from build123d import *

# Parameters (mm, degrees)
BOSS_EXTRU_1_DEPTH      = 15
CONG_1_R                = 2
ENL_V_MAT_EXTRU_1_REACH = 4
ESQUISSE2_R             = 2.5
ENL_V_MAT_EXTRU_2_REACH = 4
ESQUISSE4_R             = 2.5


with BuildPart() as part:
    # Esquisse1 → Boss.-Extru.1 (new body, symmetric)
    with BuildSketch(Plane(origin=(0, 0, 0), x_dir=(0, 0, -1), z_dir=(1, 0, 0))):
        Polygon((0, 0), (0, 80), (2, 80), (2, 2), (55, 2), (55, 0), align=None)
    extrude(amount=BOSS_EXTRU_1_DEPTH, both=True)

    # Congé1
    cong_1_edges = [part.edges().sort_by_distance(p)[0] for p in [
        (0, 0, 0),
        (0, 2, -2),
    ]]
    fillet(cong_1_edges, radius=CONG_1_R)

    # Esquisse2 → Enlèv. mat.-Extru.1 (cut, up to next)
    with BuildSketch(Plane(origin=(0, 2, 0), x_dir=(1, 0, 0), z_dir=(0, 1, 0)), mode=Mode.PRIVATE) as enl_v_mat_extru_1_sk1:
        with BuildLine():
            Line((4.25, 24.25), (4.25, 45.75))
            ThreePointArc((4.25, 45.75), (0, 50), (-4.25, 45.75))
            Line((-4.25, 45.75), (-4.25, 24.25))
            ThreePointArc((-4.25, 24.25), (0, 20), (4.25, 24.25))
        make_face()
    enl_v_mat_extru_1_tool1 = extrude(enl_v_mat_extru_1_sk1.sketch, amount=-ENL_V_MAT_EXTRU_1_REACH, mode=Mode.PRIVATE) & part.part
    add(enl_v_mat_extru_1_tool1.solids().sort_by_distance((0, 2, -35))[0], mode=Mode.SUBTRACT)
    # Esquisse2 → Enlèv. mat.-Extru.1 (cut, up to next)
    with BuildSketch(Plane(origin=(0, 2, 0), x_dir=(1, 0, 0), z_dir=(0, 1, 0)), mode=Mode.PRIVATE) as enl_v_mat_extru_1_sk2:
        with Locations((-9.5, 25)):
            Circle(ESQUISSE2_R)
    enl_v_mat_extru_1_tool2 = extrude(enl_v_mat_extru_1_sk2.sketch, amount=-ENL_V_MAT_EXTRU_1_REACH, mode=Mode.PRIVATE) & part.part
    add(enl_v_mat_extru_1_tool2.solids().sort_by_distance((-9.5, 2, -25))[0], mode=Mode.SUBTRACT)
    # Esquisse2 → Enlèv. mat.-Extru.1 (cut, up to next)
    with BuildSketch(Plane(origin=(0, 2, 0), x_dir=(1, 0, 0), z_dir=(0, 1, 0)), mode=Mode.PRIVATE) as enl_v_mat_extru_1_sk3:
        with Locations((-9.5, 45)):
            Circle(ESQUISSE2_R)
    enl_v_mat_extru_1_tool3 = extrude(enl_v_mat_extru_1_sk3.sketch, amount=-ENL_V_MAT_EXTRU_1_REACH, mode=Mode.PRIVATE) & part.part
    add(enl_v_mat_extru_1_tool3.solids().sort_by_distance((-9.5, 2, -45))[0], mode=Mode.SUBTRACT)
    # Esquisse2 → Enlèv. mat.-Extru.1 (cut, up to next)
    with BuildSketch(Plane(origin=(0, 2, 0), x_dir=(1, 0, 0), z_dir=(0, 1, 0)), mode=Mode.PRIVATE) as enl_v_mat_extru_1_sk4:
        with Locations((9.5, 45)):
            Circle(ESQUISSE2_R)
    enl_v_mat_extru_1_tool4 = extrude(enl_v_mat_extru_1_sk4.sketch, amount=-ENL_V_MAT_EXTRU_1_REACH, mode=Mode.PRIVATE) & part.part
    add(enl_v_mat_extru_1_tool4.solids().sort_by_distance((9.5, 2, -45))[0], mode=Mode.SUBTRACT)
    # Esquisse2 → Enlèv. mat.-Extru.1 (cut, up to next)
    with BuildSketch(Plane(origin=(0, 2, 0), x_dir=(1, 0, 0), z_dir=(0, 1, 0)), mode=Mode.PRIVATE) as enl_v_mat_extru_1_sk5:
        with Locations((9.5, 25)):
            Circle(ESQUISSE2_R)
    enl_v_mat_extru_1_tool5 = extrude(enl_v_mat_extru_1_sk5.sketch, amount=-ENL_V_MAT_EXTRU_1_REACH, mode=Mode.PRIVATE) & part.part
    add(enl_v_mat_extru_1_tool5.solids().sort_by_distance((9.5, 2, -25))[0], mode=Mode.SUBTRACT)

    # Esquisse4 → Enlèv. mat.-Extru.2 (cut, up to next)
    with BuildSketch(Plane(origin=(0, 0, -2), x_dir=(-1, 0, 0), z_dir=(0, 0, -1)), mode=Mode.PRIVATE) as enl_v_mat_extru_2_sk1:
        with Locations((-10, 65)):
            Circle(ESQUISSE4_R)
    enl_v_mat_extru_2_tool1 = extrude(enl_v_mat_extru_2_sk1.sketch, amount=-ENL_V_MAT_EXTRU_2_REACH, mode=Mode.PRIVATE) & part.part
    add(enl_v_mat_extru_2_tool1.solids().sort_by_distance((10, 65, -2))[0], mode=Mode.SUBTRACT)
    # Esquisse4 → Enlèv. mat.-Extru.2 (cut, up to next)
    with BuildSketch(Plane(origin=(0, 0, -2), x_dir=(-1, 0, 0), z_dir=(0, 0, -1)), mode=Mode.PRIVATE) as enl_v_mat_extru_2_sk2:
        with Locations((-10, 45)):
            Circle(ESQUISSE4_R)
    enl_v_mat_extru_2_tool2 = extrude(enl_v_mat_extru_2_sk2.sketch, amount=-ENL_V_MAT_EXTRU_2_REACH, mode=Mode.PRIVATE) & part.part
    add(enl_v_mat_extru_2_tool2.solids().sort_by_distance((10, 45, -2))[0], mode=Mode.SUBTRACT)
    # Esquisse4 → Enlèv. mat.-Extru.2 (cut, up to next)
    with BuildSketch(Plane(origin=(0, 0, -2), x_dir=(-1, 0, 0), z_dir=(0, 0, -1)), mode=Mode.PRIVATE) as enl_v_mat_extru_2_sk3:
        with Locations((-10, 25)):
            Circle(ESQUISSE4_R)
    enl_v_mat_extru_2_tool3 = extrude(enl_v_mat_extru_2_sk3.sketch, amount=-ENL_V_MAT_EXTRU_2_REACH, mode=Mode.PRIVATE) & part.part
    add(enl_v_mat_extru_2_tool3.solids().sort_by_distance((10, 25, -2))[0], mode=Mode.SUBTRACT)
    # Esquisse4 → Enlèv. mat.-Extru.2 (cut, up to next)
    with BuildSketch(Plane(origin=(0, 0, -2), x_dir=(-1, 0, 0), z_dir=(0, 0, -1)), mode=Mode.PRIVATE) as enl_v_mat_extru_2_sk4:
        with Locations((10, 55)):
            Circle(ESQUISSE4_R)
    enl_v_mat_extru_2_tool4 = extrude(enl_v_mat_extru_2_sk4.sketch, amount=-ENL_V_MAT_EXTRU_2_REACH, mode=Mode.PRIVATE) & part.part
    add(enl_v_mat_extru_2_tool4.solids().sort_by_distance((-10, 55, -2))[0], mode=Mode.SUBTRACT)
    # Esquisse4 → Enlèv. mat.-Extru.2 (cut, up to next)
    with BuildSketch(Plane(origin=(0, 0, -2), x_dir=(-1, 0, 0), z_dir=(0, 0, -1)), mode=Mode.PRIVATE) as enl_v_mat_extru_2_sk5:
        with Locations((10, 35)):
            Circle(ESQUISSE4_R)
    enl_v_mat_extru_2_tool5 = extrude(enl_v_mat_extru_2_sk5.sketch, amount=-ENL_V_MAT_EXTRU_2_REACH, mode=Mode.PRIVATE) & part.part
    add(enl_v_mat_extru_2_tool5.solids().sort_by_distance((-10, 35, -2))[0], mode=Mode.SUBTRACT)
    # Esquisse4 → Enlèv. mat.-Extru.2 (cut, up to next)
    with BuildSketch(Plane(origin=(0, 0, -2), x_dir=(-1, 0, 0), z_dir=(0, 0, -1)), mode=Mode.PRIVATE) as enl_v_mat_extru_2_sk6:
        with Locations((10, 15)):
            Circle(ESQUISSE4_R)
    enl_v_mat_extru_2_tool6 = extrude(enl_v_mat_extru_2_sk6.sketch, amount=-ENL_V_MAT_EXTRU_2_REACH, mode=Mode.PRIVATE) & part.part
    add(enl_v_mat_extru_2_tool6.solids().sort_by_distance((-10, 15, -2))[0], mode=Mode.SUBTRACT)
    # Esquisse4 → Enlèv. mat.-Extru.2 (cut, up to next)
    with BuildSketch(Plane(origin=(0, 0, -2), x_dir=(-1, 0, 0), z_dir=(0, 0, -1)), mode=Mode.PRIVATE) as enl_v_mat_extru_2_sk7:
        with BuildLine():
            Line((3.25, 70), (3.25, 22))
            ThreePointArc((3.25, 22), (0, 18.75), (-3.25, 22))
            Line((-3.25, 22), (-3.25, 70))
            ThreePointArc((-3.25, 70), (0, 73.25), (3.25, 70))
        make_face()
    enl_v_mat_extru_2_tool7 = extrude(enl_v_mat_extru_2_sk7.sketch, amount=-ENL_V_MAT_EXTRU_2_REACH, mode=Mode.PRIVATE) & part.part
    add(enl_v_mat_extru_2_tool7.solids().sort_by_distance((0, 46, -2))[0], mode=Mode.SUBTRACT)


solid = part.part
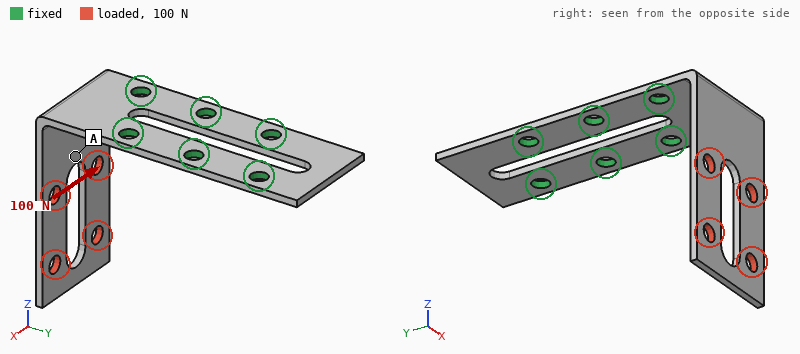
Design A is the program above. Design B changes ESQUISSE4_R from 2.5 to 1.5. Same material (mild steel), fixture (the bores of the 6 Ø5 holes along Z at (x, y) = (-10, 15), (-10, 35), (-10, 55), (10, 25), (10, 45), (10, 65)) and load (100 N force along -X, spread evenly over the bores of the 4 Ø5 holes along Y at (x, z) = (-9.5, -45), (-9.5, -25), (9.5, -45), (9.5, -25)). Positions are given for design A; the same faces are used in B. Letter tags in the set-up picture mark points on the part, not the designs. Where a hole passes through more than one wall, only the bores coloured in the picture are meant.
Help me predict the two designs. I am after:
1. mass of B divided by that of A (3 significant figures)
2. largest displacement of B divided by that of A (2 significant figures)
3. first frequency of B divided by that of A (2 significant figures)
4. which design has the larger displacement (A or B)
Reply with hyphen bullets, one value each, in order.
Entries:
- 1.02
- 1.1
- 0.97
- B
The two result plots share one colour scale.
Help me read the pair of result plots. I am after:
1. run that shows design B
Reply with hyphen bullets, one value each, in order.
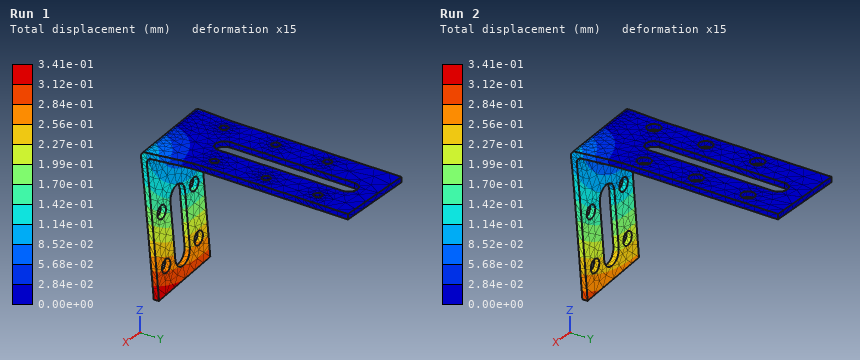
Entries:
- Run 1
